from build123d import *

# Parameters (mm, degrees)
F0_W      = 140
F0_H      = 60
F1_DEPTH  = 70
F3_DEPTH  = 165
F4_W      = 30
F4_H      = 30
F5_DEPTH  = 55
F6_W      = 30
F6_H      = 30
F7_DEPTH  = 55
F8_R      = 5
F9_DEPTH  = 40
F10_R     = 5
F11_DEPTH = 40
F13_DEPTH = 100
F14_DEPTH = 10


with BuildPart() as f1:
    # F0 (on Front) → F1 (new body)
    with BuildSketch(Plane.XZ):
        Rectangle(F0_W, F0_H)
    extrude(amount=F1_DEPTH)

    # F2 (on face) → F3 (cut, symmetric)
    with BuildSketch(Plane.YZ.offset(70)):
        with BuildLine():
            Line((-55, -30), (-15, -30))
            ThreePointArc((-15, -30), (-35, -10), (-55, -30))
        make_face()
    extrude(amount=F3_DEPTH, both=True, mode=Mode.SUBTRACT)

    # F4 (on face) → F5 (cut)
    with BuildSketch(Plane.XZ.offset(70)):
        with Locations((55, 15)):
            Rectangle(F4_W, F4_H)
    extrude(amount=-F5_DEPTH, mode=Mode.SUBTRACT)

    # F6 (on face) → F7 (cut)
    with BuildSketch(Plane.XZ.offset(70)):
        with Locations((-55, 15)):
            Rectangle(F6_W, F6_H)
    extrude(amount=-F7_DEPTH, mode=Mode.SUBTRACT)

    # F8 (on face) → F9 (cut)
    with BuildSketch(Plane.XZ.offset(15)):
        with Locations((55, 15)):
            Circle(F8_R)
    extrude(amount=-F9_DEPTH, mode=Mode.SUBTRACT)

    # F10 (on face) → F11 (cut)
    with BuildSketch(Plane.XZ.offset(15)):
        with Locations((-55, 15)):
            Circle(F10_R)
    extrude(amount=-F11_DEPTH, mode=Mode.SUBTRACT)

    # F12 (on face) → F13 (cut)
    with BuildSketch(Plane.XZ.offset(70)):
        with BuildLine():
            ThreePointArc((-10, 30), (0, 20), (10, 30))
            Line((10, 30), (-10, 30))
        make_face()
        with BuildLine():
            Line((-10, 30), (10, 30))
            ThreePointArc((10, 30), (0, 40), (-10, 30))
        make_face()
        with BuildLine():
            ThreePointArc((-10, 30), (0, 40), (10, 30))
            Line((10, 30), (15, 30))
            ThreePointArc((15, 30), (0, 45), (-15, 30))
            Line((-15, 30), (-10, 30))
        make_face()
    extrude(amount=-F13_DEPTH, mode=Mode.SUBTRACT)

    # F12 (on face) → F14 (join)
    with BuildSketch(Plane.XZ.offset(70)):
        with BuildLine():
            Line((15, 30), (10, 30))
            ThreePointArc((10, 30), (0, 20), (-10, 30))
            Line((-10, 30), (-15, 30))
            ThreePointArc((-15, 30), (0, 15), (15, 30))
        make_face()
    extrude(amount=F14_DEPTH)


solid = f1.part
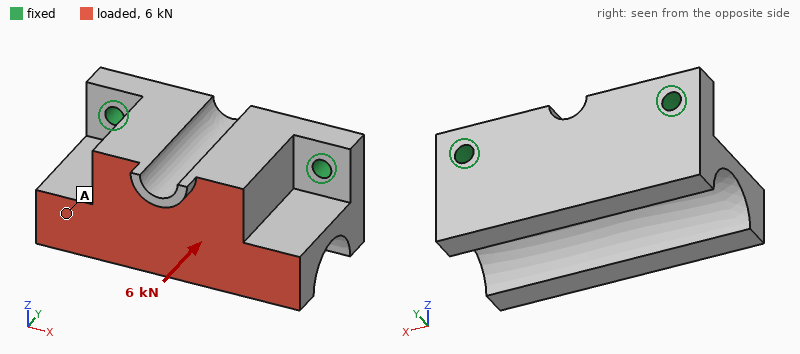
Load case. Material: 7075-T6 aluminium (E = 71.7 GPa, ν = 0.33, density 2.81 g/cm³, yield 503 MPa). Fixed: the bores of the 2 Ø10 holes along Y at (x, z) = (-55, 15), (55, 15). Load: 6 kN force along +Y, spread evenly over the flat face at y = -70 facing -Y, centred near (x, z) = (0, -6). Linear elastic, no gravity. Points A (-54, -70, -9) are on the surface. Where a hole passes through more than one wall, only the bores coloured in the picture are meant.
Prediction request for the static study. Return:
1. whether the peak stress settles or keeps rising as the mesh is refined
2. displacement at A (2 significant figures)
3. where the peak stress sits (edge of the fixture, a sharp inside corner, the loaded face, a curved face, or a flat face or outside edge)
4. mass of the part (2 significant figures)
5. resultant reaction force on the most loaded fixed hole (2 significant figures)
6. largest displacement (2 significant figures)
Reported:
keeps rising
50 µm
edge of the fixture
1.1 kg
3.1 kN
59 µm
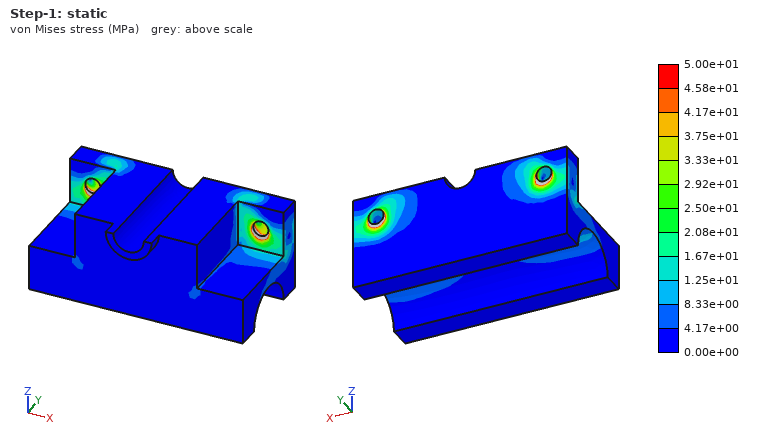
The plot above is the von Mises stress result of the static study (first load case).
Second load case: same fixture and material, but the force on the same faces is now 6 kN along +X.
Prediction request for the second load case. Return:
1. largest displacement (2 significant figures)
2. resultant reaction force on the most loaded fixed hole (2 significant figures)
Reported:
19 µm
4.8 kN
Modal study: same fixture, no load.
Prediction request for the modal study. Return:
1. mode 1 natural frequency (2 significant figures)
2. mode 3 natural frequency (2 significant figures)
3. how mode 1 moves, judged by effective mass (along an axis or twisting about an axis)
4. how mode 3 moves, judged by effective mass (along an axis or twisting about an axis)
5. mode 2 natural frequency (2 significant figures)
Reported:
1400 Hz
4800 Hz
along Z
along X
4600 Hz
